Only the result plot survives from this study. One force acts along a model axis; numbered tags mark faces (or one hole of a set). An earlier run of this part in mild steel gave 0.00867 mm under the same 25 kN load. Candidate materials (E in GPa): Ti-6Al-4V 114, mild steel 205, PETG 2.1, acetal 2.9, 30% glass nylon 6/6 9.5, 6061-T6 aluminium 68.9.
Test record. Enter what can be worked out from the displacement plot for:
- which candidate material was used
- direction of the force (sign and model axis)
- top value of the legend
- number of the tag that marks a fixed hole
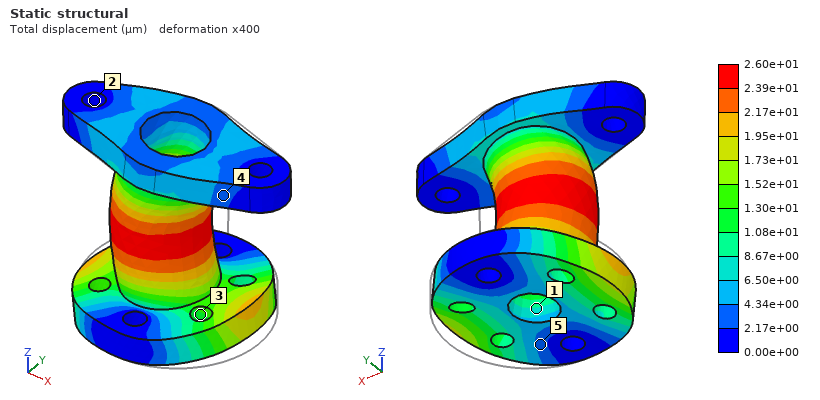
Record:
6061-T6 aluminium
-X
2.60e+01 µm
2
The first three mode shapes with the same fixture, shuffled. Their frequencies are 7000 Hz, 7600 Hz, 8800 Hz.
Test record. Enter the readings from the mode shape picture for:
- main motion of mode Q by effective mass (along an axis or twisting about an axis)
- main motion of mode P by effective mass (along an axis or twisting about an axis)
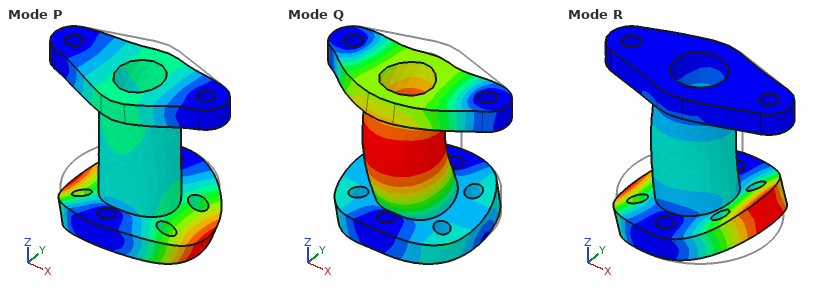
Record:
along Y
along Z
